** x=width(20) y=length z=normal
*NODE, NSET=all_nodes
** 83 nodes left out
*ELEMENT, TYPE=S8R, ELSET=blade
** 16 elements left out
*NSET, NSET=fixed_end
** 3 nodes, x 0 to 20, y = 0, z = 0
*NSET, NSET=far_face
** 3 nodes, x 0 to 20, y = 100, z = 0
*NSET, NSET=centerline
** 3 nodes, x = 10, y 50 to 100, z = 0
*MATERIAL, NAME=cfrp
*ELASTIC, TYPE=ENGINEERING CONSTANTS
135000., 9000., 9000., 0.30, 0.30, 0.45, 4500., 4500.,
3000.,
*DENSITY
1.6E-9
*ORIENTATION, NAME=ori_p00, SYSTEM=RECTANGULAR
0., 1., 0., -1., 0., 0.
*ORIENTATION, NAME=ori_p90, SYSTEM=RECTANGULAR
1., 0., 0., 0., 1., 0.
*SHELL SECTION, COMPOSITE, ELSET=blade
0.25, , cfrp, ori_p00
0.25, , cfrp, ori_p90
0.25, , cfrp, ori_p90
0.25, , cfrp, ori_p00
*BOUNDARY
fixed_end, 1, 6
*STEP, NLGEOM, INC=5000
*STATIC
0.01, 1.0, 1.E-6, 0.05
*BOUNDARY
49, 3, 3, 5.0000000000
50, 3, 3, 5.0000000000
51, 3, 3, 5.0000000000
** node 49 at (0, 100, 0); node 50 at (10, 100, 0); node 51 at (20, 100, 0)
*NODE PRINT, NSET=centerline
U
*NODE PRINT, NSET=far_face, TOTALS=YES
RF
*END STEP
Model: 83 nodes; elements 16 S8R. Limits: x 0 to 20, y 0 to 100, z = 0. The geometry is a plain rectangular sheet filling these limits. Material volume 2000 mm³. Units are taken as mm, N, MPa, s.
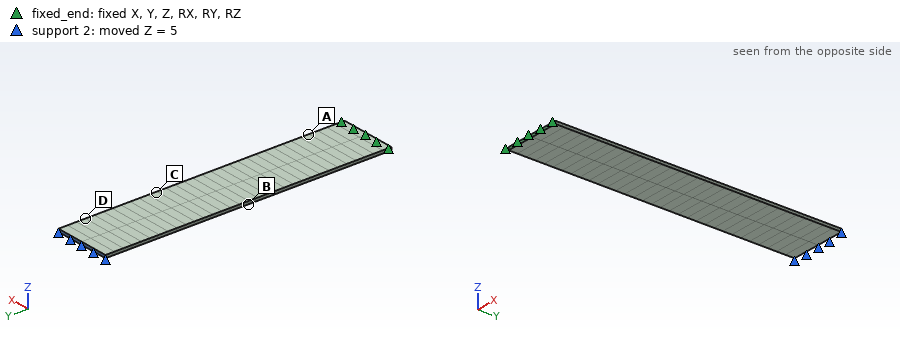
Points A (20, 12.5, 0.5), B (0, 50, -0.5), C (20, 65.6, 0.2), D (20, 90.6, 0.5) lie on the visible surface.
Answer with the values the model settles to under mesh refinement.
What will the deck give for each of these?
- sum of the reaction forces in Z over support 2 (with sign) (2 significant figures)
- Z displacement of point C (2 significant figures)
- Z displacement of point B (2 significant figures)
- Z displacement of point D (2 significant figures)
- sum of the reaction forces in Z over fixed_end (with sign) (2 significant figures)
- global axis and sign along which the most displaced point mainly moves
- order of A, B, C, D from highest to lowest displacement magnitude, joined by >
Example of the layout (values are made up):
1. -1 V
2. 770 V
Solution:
1. 3.0 N
2. 2.5 mm
3. 1.6 mm
4. 4.3 mm
5. -3.0 N
6. +Z
7. D > C > B > A
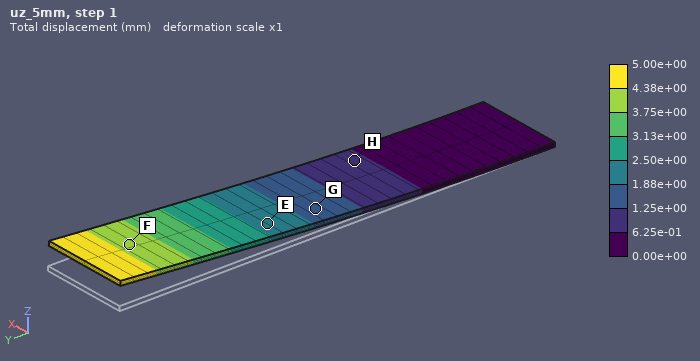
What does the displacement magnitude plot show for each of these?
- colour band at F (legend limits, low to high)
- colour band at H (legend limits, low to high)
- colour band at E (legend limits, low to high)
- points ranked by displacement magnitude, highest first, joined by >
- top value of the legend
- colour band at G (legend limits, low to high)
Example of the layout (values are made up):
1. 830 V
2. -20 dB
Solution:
1. 3.75e+00 to 4.38e+00 mm
2. 6.25e-01 to 1.25e+00 mm
3. 1.88e+00 to 2.50e+00 mm
4. F > E > G > H
5. 5.00e+00 mm
6. 1.25e+00 to 1.88e+00 mm
